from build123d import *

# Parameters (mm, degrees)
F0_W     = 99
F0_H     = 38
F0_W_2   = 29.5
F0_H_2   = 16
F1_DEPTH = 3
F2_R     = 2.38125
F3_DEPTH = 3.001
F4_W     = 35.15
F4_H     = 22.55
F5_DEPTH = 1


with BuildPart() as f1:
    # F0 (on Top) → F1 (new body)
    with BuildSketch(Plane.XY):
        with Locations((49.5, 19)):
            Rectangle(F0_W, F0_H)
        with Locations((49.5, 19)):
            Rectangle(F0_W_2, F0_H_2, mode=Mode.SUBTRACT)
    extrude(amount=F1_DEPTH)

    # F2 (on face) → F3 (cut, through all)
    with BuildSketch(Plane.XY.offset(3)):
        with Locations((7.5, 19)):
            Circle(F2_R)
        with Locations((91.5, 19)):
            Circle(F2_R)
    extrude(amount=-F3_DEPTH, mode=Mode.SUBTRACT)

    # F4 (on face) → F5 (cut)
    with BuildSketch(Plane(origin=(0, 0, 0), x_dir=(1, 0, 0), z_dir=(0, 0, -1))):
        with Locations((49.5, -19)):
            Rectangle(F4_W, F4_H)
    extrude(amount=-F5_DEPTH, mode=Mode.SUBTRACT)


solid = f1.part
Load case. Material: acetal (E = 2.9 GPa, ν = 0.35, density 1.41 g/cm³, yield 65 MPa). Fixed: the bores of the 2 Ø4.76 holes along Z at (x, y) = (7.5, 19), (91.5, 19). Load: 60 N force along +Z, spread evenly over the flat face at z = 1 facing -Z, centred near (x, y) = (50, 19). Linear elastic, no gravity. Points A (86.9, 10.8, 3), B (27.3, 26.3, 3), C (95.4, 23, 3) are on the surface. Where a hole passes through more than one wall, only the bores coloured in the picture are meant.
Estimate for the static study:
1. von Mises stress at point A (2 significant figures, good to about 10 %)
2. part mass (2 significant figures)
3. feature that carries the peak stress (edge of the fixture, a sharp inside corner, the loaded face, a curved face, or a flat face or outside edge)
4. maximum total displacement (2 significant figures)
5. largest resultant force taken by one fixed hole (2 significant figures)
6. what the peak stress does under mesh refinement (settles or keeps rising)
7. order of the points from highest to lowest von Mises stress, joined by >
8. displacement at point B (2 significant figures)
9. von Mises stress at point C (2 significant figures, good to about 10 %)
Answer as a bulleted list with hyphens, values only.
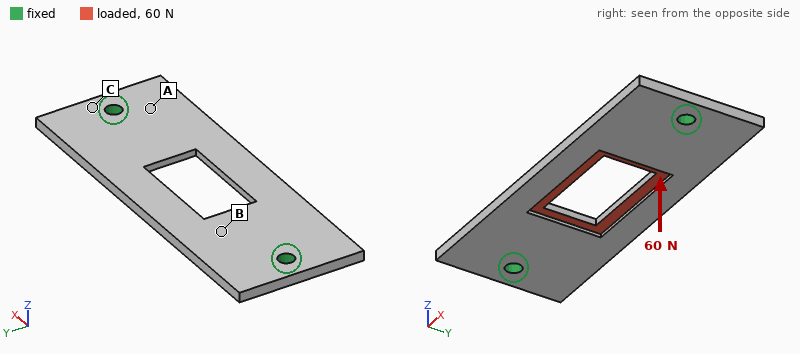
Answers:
- 7.6 MPa
- 13 g
- edge of the fixture
- 0.96 mm
- 34 N
- keeps rising
- A > C > B
- 0.45 mm
- 3.8 MPa
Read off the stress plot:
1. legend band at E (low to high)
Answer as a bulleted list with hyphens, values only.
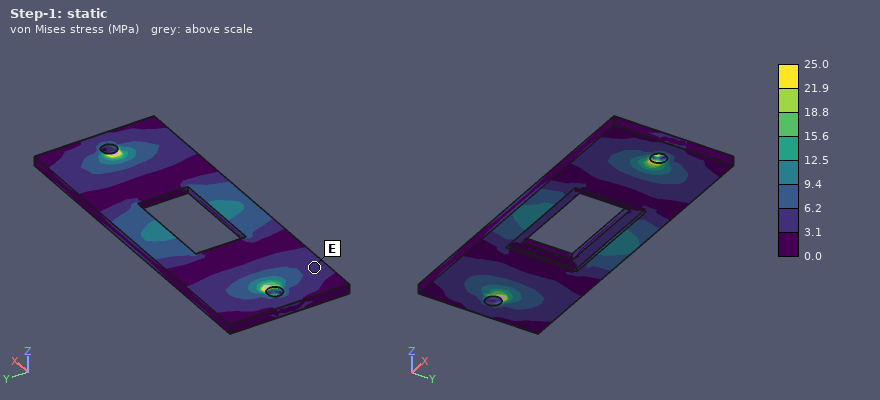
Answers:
- 3.1 to 6.2 MPa
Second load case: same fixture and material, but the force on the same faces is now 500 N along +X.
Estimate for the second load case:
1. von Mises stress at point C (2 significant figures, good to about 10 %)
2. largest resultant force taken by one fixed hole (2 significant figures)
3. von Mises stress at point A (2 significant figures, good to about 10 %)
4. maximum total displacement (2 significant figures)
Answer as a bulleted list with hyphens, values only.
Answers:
- 3.3 MPa
- 250 N
- 2.9 MPa
- 61 µm
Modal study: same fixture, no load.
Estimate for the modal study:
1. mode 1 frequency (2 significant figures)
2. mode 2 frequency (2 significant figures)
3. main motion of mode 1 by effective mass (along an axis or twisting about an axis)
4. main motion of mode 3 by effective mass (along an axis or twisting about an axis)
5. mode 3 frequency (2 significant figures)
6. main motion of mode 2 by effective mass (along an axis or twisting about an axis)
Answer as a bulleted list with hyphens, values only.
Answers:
- 640 Hz
- 760 Hz
- along Z
- twisting about Y
- 1400 Hz
- twisting about X
